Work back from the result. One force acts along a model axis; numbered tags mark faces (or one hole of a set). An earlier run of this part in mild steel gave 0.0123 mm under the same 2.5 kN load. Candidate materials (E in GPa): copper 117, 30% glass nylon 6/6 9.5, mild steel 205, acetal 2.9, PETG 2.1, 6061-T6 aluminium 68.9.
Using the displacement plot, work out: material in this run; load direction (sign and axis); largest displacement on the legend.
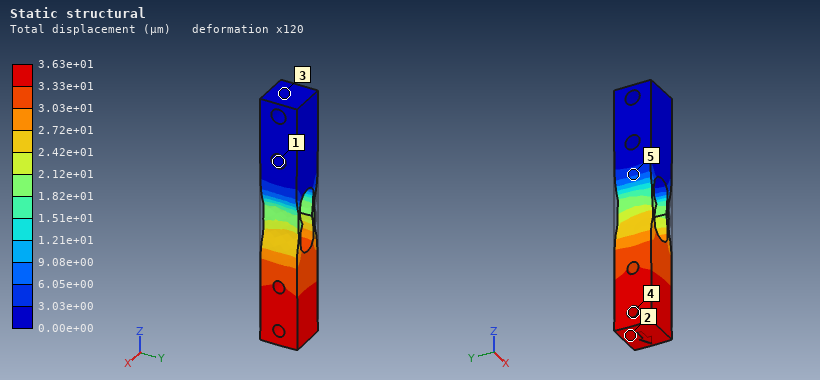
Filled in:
6061-T6 aluminium
-Z
3.63e+01 µm
